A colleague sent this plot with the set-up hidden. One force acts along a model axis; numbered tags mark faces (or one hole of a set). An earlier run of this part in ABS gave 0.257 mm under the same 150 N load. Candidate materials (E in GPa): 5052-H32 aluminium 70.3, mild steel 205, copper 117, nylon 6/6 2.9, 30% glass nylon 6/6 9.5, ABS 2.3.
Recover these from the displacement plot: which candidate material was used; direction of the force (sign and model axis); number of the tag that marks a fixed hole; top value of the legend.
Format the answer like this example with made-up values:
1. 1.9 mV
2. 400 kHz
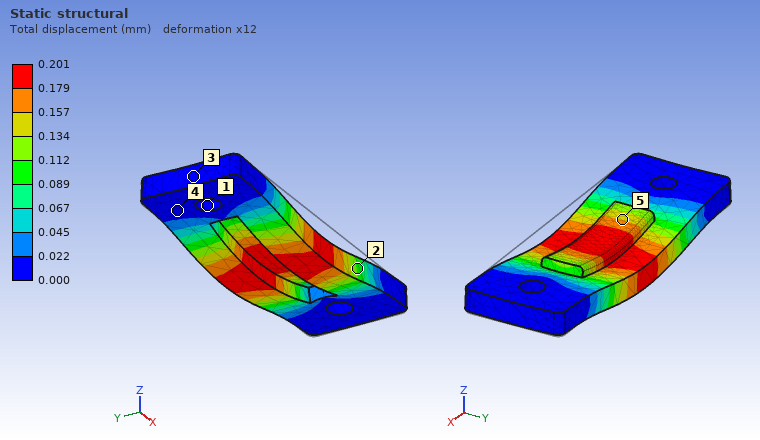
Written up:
1. nylon 6/6
2. -Z
3. 1
4. 0.201 mm
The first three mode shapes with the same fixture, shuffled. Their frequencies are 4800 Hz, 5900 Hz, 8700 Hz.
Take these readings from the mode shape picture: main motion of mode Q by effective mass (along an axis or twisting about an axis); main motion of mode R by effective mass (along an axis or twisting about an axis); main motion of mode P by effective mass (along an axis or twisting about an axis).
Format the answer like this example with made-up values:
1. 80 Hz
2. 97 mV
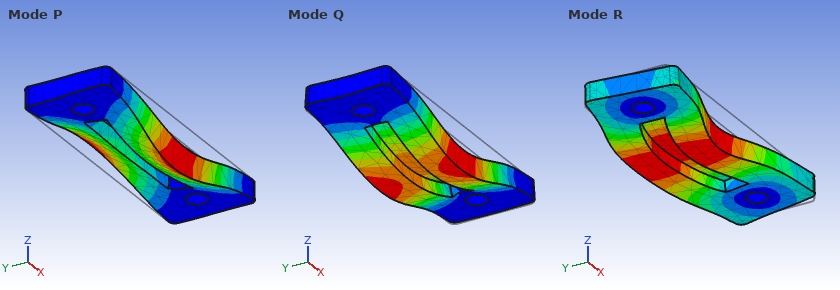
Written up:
1. along Z
2. along Y
3. twisting about X
